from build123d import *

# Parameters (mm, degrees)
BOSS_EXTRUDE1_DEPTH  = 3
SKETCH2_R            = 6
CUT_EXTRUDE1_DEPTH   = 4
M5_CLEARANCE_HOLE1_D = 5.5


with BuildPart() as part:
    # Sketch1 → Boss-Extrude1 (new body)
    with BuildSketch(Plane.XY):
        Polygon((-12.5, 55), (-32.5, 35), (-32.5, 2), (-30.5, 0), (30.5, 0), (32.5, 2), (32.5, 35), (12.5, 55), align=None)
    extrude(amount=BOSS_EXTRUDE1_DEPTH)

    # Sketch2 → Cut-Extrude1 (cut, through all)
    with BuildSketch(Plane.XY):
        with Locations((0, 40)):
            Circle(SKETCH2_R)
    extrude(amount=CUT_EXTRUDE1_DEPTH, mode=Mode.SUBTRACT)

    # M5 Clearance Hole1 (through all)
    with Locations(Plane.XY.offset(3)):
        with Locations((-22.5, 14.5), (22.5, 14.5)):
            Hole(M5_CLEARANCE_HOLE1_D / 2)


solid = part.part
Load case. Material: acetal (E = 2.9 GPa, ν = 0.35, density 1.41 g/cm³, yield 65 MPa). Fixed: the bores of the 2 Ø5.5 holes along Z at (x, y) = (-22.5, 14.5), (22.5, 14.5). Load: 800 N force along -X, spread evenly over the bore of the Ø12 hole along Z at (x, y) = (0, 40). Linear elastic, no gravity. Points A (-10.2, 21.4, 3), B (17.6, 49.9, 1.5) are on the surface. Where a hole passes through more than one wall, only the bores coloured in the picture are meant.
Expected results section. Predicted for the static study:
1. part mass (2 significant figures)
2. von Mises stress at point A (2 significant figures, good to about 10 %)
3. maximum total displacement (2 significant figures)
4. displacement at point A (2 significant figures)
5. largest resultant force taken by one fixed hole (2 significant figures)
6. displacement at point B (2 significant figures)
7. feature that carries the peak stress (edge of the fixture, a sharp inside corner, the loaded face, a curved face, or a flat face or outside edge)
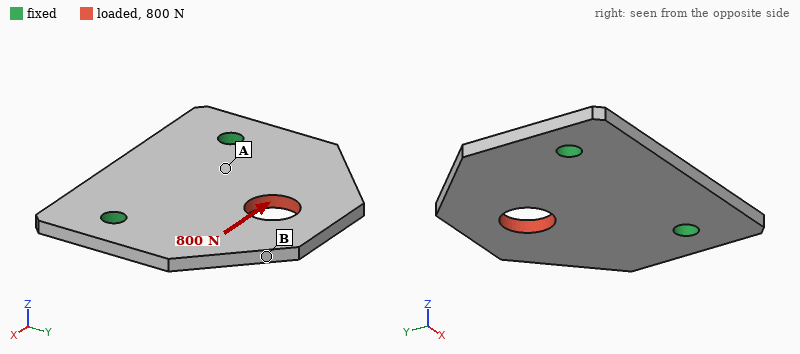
13 g
8.6 MPa
0.22 mm
0.045 mm
580 N
0.20 mm
edge of the fixture
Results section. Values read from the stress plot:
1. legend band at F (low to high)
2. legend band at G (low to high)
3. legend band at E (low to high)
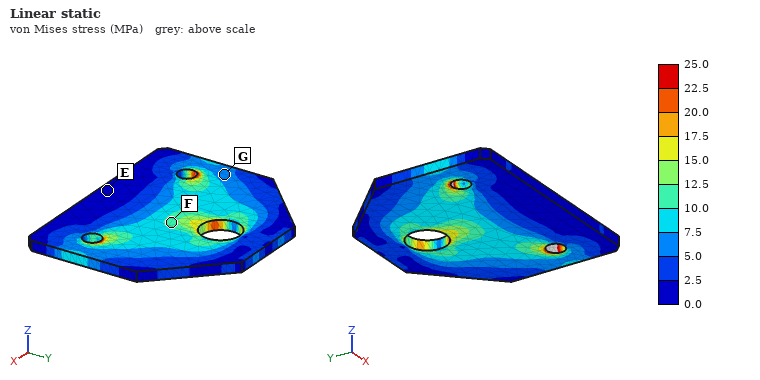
10.0 to 12.5 MPa
5.0 to 7.5 MPa
0.0 to 2.5 MPa
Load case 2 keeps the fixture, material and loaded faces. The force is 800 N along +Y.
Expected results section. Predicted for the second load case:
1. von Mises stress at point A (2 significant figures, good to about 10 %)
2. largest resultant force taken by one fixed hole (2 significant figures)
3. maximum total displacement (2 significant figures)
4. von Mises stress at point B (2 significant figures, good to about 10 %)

5.7 MPa
420 N
0.13 mm
2.5 MPa
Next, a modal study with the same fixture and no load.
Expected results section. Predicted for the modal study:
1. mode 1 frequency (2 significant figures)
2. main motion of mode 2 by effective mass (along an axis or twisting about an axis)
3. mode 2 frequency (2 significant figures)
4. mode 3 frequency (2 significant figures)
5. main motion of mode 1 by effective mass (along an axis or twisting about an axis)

520 Hz
twisting about Y
1200 Hz
2000 Hz
along Z
